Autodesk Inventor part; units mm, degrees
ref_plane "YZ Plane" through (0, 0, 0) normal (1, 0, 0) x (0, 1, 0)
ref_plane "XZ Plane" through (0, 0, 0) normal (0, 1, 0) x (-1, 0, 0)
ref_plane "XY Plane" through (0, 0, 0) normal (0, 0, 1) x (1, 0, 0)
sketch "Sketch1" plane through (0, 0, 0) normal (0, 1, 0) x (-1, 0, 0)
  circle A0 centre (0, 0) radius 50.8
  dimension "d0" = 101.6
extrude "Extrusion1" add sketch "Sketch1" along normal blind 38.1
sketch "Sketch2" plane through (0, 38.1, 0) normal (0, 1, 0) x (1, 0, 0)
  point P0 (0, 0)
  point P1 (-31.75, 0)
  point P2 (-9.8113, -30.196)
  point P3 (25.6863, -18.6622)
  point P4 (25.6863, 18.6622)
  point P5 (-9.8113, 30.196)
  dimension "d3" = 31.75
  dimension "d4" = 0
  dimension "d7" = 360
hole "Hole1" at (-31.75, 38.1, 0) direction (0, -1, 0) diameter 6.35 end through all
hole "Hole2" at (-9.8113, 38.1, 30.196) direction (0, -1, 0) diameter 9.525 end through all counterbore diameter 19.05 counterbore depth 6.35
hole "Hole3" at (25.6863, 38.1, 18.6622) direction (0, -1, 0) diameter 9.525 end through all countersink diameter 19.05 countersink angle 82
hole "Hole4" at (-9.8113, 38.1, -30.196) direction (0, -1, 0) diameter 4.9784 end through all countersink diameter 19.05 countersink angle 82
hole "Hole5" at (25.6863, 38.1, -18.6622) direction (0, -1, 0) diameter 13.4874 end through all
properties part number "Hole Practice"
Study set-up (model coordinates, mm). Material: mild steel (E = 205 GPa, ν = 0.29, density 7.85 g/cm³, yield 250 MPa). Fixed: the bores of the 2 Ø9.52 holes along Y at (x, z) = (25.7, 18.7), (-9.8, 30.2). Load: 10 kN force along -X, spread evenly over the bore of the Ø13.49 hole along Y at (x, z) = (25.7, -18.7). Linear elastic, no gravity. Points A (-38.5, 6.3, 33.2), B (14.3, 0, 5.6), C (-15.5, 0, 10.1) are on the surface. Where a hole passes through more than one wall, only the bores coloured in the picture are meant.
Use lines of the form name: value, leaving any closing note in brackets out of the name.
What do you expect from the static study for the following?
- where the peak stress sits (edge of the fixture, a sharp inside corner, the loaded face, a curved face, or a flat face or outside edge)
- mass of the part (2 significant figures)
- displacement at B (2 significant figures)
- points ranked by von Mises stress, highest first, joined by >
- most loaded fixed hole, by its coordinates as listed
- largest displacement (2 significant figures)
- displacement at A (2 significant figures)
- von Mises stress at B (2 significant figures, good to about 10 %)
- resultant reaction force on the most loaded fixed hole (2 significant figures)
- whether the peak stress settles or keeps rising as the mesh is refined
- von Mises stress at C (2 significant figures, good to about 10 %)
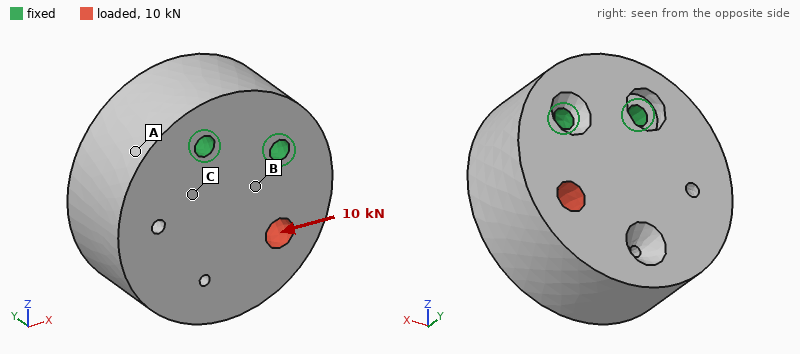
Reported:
where the peak stress sits: edge of the fixture
mass of the part: 2.3 kg
displacement at B: 1.3 µm
points ranked by von Mises stress, highest first, joined by >: B > C > A
most loaded fixed hole, by its coordinates as listed: (25.7, 18.7)
largest displacement: 5.7 µm
displacement at A: 2.2 µm
von Mises stress at B: 13 MPa
resultant reaction force on the most loaded fixed hole: 12 kN
whether the peak stress settles or keeps rising as the mesh is refined: keeps rising
von Mises stress at C: 6.3 MPa
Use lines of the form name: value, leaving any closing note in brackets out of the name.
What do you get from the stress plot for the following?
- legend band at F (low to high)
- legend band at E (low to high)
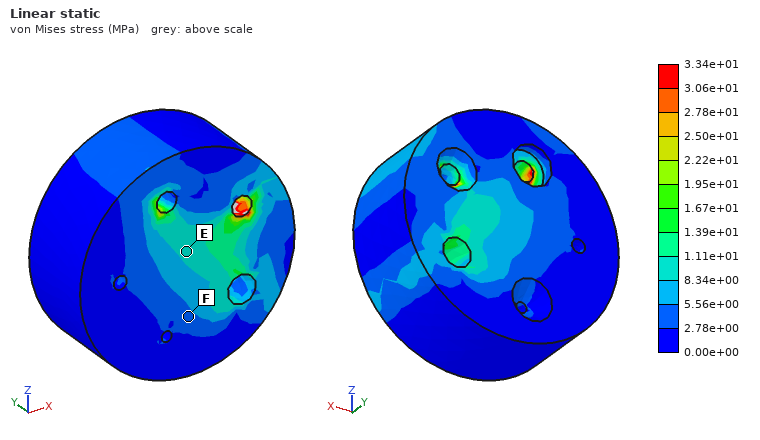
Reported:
legend band at F: 2.78e+00 to 5.56e+00 MPa
legend band at E: 8.34e+00 to 1.11e+01 MPa
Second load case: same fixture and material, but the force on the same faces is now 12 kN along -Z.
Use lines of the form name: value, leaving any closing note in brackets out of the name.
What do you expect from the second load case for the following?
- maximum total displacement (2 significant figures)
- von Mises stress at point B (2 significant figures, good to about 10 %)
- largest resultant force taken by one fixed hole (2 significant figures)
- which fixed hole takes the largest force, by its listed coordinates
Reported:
maximum total displacement: 2.7 µm
von Mises stress at point B: 5.3 MPa
largest resultant force taken by one fixed hole: 11 kN
which fixed hole takes the largest force, by its listed coordinates: (25.7, 18.7)
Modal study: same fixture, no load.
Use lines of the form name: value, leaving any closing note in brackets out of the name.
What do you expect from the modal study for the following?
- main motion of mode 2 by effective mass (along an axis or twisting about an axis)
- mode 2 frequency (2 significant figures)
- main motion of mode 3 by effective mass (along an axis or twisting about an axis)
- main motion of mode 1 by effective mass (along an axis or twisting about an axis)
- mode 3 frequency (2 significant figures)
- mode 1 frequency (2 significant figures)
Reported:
main motion of mode 2 by effective mass: along X
mode 2 frequency: 6000 Hz
main motion of mode 3 by effective mass: twisting about Z
main motion of mode 1 by effective mass: along Y
mode 3 frequency: 8100 Hz
mode 1 frequency: 4400 Hz
